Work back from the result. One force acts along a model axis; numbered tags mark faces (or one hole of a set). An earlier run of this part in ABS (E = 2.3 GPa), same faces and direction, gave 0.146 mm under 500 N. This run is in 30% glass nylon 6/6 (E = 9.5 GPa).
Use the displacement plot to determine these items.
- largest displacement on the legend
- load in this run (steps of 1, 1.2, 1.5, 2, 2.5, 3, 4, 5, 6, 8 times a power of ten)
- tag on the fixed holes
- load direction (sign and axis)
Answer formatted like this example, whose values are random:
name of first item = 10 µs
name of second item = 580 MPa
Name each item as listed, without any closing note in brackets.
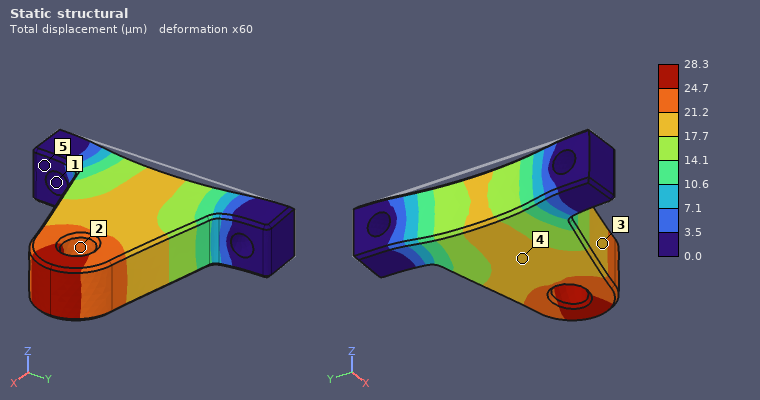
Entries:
largest displacement on the legend = 28.3 µm
load in this run = 400 N
tag on the fixed holes = 1
load direction = +X
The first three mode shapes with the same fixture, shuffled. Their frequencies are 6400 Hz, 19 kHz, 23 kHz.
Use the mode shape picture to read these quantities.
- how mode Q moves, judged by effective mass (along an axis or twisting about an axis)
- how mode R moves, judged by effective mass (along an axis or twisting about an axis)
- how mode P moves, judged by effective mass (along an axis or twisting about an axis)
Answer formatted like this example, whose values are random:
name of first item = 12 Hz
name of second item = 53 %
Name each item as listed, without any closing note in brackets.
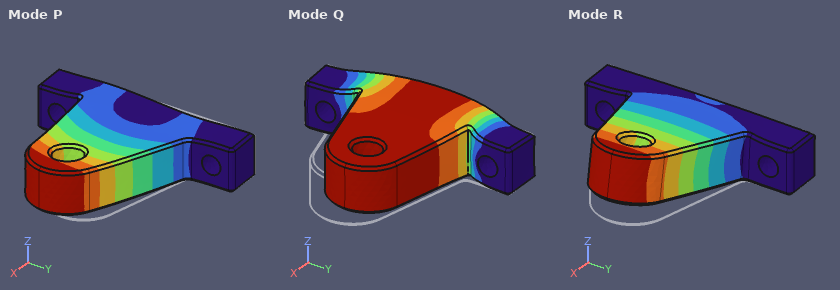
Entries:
how mode Q moves, judged by effective mass = along X
how mode R moves, judged by effective mass = along Z
how mode P moves, judged by effective mass = along Y
